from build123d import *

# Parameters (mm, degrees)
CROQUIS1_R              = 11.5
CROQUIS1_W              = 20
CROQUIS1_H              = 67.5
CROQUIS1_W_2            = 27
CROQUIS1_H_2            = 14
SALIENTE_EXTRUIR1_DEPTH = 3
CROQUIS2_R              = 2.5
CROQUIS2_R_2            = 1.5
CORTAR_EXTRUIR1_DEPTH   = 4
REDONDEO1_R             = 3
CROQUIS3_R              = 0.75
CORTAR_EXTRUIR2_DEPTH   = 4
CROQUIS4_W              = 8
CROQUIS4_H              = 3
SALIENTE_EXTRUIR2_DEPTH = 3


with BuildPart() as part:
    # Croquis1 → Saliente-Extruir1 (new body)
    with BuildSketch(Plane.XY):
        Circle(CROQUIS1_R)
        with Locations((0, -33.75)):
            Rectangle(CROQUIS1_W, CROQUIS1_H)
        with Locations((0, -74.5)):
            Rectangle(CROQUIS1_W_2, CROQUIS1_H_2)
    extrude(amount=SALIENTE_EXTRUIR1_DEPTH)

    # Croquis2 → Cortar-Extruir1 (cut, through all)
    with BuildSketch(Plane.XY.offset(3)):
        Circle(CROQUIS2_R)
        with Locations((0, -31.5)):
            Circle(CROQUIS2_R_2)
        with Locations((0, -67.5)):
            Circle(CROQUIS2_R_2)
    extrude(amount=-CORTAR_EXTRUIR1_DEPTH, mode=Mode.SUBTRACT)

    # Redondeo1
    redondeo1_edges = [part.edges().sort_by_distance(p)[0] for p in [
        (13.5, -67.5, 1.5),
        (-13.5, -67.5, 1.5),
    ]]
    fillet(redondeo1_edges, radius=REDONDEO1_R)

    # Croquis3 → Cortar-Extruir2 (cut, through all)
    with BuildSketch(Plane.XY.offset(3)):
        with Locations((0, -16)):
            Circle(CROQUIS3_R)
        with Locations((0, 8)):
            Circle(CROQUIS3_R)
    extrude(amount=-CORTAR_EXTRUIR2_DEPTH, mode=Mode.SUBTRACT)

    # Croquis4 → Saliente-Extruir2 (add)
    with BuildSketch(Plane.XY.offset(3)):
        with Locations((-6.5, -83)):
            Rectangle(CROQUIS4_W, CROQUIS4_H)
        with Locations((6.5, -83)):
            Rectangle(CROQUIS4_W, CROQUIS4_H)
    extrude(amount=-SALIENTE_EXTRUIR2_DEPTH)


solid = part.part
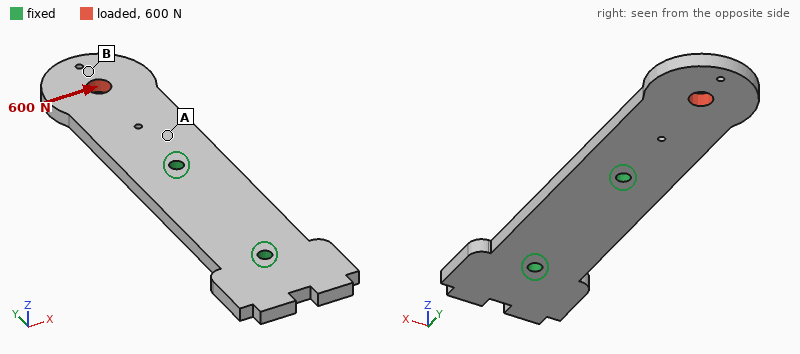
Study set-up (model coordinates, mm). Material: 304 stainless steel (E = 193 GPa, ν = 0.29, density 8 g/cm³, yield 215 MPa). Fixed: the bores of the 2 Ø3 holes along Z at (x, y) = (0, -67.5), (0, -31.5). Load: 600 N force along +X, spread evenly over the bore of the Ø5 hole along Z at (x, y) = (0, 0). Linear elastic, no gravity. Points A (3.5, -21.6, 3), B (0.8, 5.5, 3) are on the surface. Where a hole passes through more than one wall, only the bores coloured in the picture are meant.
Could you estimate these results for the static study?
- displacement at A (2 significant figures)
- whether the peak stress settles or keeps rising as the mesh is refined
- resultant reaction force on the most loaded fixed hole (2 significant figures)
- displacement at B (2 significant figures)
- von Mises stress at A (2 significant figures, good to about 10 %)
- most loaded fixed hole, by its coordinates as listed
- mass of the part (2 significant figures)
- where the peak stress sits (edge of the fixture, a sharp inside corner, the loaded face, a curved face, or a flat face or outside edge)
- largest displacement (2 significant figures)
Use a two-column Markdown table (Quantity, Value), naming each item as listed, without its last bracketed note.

| Quantity | Value |
|---|---|
| displacement at A | 10 µm |
| whether the peak stress settles or keeps rising as the mesh is refined | keeps rising |
| resultant reaction force on the most loaded fixed hole | 1.0 kN |
| displacement at B | 48 µm |
| von Mises stress at A | 31 MPa |
| most loaded fixed hole, by its coordinates as listed | (0, -31.5) |
| mass of the part | 47 g |
| where the peak stress sits | edge of the fixture |
| largest displacement | 56 µm |
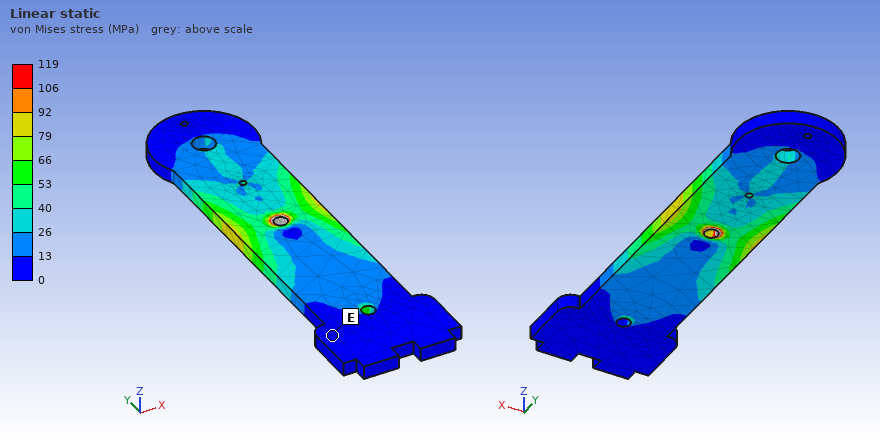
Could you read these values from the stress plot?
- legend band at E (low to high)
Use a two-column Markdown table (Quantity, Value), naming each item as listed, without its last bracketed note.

| Quantity | Value |
|---|---|
| legend band at E | 0 to 13 MPa |
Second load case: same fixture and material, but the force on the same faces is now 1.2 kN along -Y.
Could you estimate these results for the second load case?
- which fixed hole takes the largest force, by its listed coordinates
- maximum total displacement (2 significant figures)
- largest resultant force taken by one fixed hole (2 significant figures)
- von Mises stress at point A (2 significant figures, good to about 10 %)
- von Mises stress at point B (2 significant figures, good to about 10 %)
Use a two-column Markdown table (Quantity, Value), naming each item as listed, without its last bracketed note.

| Quantity | Value |
|---|---|
| which fixed hole takes the largest force, by its listed coordinates | (0, -31.5) |
| maximum total displacement | 4.8 µm |
| largest resultant force taken by one fixed hole | 1.0 kN |
| von Mises stress at point A | 23 MPa |
| von Mises stress at point B | 15 MPa |
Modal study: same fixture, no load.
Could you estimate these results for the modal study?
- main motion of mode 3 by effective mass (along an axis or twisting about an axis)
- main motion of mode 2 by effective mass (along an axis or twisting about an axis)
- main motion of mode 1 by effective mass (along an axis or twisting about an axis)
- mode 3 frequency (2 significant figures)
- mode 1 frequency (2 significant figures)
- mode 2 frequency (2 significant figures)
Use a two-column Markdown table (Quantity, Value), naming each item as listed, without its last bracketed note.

| Quantity | Value |
|---|---|
| main motion of mode 3 by effective mass | along X |
| main motion of mode 2 by effective mass | twisting about Y |
| main motion of mode 1 by effective mass | along Z |
| mode 3 frequency | 5700 Hz |
| mode 1 frequency | 1400 Hz |
| mode 2 frequency | 5000 Hz |
